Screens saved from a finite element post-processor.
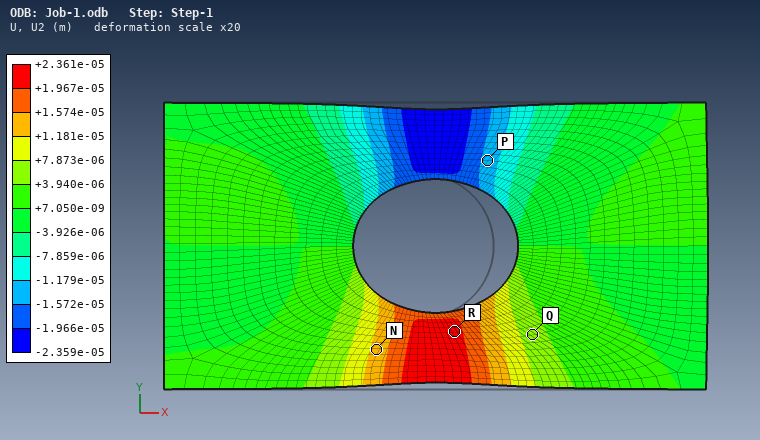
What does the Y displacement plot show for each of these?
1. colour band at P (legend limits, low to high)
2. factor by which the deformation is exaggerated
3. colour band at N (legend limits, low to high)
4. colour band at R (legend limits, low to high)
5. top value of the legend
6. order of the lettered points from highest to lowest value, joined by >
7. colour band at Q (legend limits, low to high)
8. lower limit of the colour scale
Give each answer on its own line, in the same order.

-1.572e-05 to -1.179e-05 m
20
+1.181e-05 to +1.574e-05 m
+1.967e-05 to +2.361e-05 m
+2.361e-05 m
R > N > Q > P
+3.940e-06 to +7.873e-06 m
-2.359e-05 m
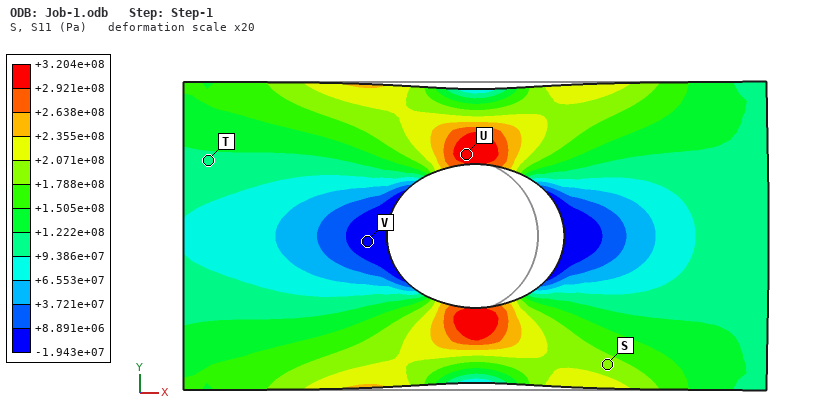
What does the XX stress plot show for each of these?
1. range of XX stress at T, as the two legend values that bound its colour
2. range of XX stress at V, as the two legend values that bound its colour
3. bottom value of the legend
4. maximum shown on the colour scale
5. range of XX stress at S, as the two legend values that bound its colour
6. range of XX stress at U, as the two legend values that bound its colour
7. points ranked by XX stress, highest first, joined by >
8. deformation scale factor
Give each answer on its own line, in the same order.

+9.386e+07 to +1.222e+08 Pa
-1.943e+07 to +8.891e+06 Pa
-1.943e+07 Pa
+3.204e+08 Pa
+1.788e+08 to +2.071e+08 Pa
+2.921e+08 to +3.204e+08 Pa
U > S > T > V
20
